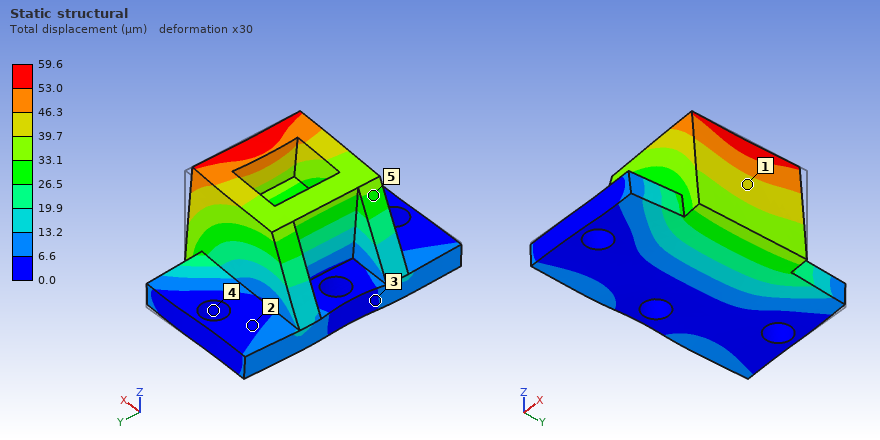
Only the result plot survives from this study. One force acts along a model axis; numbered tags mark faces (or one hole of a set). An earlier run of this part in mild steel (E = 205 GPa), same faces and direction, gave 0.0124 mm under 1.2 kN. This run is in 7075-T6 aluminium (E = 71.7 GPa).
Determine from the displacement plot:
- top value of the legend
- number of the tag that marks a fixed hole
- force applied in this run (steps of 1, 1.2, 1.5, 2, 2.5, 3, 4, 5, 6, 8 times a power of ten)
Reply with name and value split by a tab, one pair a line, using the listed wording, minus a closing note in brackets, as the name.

top value of the legend	59.6 µm
number of the tag that marks a fixed hole	4
force applied in this run	2 kN
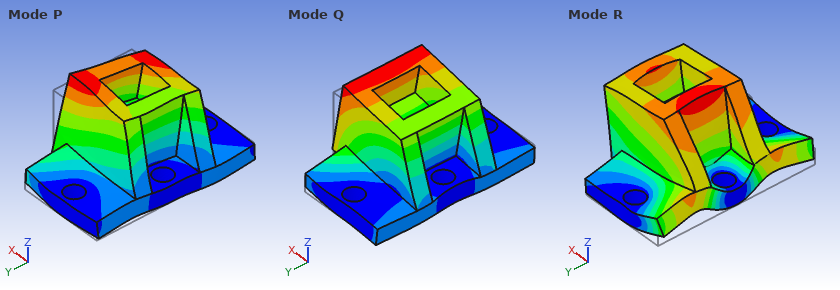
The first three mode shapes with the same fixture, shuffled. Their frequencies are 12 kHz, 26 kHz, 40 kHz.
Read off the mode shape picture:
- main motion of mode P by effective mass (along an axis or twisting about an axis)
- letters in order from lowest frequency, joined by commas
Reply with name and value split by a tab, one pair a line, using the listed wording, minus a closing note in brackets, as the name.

main motion of mode P by effective mass	along Y
letters in order from lowest frequency, joined by commas	Q, P, R
